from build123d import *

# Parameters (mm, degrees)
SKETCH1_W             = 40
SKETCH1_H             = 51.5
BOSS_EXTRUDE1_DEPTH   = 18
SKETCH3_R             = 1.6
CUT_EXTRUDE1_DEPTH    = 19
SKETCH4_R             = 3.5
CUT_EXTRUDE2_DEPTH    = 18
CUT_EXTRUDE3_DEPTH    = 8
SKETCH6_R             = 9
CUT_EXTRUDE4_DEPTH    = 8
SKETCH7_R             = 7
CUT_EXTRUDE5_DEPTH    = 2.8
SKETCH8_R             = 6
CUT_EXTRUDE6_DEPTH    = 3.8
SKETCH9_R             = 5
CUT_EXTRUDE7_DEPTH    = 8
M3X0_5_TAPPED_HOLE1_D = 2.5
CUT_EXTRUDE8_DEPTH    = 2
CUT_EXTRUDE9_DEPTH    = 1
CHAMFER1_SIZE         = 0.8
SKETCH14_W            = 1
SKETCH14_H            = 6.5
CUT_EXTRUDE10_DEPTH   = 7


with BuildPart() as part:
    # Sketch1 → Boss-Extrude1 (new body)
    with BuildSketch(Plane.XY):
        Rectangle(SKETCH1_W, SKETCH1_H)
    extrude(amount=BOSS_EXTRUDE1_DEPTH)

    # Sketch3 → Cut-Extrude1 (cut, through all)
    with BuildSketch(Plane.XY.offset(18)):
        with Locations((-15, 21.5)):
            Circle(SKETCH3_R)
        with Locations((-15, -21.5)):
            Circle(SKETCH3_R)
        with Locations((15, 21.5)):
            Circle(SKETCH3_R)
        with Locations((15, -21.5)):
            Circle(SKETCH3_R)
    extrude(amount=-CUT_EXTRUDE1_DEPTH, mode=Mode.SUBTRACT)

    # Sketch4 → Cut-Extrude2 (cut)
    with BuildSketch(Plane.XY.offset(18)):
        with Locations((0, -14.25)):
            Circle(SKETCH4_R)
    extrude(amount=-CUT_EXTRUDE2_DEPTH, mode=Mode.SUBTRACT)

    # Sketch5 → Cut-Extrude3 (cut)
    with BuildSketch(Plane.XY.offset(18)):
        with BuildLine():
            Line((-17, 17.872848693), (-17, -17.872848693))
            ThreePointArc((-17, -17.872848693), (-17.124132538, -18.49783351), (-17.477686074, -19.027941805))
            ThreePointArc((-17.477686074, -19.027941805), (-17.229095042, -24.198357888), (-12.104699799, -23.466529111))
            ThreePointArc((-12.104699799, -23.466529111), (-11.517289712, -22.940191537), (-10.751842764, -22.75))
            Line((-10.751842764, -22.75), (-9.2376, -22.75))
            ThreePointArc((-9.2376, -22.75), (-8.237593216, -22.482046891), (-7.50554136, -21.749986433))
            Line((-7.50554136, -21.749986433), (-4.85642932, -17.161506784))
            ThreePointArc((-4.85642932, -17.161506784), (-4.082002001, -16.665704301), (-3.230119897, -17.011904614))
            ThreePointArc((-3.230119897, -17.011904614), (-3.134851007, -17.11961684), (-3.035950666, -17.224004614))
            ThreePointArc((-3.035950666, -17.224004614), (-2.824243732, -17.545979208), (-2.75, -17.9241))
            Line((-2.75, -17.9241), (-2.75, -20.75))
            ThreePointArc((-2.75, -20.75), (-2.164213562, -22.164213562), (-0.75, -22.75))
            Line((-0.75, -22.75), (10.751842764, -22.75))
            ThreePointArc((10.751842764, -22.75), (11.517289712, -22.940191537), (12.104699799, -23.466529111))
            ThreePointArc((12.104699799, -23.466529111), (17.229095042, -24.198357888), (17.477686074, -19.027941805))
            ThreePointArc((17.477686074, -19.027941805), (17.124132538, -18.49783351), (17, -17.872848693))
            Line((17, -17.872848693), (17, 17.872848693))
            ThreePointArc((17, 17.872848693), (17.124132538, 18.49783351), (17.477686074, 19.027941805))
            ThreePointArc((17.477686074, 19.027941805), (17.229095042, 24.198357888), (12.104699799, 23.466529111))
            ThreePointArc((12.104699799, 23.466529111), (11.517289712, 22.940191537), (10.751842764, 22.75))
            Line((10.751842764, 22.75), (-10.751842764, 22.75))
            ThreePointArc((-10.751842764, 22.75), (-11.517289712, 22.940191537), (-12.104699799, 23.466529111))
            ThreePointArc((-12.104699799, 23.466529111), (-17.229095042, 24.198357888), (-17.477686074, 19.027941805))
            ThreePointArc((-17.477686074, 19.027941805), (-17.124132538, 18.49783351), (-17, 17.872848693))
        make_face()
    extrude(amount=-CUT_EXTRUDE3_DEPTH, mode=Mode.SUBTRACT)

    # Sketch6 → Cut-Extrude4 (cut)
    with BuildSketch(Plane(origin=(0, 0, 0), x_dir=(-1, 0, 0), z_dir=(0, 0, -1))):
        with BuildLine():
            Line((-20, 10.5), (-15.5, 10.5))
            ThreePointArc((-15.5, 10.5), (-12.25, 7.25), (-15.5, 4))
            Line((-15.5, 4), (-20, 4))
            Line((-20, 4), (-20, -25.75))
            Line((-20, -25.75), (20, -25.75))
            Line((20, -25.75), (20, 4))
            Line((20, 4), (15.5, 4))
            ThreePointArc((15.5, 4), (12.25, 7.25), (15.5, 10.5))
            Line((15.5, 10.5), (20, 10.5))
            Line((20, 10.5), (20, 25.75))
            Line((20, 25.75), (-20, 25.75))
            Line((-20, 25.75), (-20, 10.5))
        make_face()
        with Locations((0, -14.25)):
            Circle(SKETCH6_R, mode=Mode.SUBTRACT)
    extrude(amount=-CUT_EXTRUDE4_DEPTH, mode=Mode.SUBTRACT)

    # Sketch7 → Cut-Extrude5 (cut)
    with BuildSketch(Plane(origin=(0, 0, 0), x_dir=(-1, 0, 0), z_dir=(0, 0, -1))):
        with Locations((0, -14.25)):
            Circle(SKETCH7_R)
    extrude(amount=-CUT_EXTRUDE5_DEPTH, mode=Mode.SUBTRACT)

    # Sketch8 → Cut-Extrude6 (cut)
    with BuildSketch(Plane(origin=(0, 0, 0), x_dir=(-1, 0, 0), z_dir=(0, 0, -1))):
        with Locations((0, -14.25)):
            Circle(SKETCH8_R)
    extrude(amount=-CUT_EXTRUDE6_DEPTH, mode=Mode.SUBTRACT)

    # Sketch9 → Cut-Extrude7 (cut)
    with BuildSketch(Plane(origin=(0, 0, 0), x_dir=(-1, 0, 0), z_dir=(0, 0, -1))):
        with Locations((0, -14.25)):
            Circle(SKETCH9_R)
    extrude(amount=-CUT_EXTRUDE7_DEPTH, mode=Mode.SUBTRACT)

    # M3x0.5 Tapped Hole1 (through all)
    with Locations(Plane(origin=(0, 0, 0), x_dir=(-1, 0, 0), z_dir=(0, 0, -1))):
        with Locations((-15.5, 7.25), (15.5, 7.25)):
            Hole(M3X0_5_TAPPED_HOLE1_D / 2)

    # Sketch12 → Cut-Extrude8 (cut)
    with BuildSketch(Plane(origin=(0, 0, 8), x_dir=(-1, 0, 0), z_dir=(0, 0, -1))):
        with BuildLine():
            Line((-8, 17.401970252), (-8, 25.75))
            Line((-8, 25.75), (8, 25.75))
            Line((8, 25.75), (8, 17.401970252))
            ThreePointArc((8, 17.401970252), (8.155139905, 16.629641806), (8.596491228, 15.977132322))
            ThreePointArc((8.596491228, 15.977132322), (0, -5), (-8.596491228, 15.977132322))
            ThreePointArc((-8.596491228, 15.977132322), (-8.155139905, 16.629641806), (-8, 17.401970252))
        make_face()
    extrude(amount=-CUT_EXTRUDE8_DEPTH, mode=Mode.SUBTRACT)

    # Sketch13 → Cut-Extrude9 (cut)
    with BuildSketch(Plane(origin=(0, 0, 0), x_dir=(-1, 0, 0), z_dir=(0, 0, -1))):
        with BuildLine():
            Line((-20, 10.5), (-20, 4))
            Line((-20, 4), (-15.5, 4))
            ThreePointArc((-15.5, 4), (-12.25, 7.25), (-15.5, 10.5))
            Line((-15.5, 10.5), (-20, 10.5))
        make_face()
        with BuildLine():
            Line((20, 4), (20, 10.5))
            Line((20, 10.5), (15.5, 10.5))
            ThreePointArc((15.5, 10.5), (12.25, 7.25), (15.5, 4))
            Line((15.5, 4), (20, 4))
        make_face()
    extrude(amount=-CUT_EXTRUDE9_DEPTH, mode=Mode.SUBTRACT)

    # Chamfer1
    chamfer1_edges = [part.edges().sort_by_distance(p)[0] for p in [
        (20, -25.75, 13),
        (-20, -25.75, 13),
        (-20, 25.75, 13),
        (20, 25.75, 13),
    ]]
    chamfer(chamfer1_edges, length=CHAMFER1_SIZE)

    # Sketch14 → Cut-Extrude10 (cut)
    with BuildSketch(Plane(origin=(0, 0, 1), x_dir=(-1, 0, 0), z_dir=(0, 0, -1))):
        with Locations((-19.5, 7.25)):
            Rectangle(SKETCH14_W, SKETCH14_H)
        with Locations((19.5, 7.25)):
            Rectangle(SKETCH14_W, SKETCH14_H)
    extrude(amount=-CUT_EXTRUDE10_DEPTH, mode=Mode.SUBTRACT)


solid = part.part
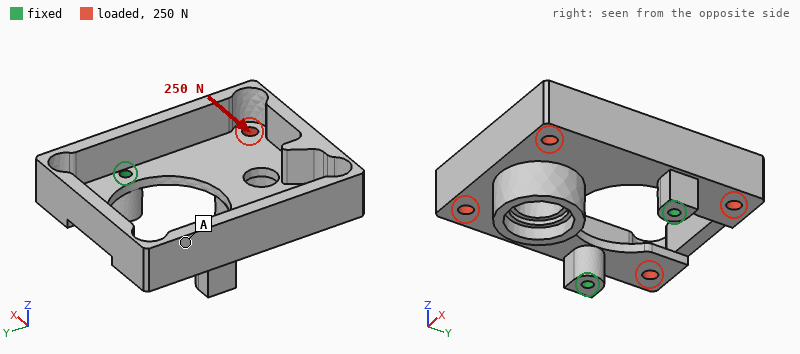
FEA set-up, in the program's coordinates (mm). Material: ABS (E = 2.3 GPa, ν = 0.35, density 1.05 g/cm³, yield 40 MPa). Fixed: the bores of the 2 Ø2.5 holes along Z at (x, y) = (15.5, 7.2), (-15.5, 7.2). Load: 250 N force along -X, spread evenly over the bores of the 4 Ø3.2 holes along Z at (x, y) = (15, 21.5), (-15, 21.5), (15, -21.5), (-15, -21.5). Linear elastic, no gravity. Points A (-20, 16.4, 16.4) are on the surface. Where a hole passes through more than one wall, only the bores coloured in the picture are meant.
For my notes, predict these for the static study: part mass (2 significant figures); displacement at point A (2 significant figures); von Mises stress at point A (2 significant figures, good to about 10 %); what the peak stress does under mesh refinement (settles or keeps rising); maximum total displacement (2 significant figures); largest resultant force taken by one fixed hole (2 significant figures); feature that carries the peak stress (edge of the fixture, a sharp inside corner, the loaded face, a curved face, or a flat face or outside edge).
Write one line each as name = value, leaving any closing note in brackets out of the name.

part mass = 8.6 g
displacement at point A = 0.11 mm
von Mises stress at point A = 2.4 MPa
what the peak stress does under mesh refinement = keeps rising
maximum total displacement = 0.29 mm
largest resultant force taken by one fixed hole = 140 N
feature that carries the peak stress = a sharp inside corner
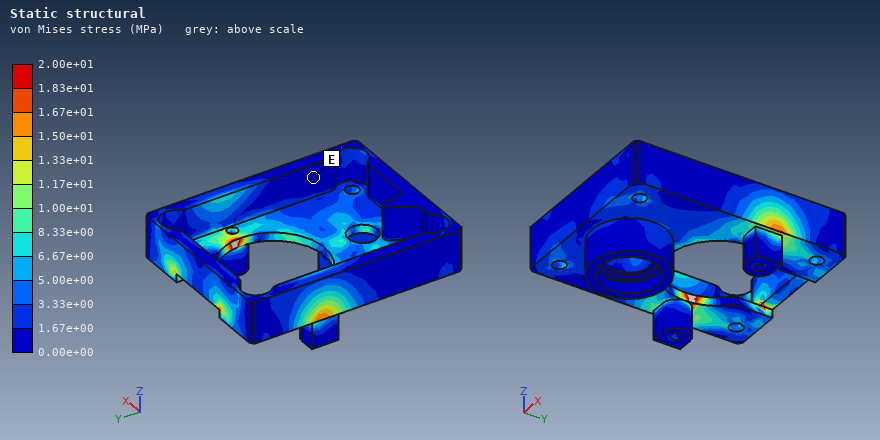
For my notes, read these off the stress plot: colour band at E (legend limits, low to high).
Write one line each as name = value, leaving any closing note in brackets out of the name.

colour band at E = 0.00e+00 to 1.67e+00 MPa
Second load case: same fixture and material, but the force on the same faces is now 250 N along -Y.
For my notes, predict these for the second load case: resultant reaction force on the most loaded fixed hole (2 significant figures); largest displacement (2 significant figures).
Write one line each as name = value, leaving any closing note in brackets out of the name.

resultant reaction force on the most loaded fixed hole = 130 N
largest displacement = 56 µm
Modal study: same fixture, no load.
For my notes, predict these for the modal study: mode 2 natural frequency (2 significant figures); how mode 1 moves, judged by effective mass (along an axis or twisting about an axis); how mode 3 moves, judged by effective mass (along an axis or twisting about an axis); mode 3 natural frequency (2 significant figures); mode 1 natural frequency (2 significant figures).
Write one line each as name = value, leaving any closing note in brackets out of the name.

mode 2 natural frequency = 1300 Hz
how mode 1 moves, judged by effective mass = along Z
how mode 3 moves, judged by effective mass = along X
mode 3 natural frequency = 2100 Hz
mode 1 natural frequency = 710 Hz
